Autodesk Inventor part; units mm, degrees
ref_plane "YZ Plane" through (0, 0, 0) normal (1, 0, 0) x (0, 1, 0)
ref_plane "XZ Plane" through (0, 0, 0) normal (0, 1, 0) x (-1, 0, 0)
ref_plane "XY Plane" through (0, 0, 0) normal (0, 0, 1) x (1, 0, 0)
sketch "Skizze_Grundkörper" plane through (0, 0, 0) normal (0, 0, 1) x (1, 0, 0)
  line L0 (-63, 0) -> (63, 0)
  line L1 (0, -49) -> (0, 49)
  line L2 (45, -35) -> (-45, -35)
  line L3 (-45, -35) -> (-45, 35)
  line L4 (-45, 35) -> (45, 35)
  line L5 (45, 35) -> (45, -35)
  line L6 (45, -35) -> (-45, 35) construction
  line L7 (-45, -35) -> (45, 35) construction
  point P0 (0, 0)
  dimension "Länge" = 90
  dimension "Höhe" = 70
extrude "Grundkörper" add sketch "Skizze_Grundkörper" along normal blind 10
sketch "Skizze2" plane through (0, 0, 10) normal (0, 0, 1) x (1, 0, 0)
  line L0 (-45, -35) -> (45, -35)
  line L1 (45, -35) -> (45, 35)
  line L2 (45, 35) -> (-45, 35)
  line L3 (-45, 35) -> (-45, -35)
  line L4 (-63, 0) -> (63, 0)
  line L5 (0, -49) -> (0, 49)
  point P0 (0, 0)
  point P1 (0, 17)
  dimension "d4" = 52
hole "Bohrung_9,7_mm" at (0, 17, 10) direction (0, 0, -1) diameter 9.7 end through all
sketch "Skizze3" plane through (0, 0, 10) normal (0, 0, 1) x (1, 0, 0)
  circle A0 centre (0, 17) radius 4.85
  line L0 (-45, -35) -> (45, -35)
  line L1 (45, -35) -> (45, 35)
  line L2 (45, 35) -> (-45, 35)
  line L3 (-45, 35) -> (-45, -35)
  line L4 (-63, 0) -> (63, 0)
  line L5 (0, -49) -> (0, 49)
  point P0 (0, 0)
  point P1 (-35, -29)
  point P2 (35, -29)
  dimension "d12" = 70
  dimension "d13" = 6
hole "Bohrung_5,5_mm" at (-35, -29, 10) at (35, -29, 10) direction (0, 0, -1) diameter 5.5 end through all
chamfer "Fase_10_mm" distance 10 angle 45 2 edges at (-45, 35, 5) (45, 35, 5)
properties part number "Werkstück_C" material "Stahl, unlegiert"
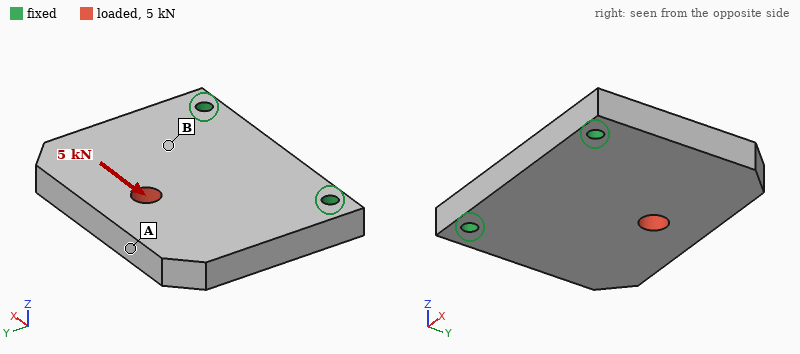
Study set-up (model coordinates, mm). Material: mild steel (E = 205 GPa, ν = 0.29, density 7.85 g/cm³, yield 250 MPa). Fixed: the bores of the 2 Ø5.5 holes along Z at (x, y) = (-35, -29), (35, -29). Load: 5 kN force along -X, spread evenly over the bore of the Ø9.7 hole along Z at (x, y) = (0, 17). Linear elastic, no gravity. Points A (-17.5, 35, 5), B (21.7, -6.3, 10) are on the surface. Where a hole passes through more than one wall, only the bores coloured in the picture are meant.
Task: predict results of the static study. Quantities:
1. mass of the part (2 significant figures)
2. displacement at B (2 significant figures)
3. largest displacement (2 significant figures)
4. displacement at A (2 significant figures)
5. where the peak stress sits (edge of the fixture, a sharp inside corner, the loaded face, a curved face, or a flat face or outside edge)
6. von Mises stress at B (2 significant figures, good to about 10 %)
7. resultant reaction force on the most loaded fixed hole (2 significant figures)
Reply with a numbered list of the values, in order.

1. 480 g
2. 3.0 µm
3. 7.5 µm
4. 7.3 µm
5. edge of the fixture
6. 13 MPa
7. 4.0 kN
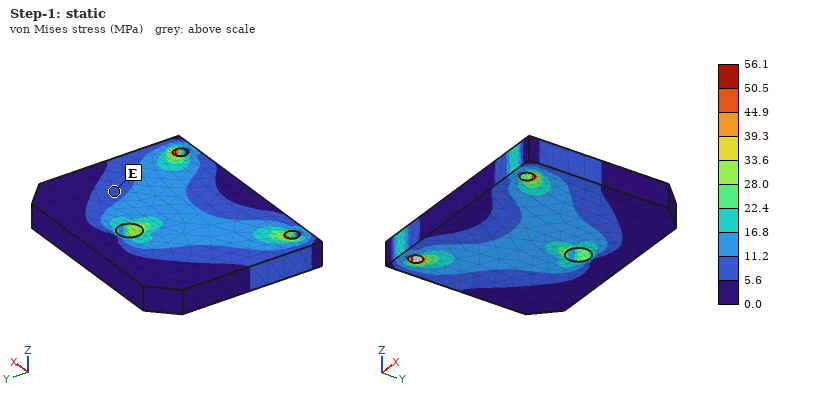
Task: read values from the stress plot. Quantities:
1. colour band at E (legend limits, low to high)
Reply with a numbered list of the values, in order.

1. 5.6 to 11.2 MPa
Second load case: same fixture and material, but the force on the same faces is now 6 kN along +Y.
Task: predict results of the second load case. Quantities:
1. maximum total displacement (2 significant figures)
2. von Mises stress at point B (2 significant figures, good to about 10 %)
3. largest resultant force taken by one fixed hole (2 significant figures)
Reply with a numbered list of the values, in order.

1. 5.1 µm
2. 12 MPa
3. 3.2 kN
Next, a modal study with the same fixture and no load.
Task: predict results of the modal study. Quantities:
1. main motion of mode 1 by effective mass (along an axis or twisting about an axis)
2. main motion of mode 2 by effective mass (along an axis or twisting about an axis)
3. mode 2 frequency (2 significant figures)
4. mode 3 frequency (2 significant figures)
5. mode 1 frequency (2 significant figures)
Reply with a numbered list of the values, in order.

1. along Z
2. twisting about Y
3. 3800 Hz
4. 7800 Hz
5. 1600 Hz
